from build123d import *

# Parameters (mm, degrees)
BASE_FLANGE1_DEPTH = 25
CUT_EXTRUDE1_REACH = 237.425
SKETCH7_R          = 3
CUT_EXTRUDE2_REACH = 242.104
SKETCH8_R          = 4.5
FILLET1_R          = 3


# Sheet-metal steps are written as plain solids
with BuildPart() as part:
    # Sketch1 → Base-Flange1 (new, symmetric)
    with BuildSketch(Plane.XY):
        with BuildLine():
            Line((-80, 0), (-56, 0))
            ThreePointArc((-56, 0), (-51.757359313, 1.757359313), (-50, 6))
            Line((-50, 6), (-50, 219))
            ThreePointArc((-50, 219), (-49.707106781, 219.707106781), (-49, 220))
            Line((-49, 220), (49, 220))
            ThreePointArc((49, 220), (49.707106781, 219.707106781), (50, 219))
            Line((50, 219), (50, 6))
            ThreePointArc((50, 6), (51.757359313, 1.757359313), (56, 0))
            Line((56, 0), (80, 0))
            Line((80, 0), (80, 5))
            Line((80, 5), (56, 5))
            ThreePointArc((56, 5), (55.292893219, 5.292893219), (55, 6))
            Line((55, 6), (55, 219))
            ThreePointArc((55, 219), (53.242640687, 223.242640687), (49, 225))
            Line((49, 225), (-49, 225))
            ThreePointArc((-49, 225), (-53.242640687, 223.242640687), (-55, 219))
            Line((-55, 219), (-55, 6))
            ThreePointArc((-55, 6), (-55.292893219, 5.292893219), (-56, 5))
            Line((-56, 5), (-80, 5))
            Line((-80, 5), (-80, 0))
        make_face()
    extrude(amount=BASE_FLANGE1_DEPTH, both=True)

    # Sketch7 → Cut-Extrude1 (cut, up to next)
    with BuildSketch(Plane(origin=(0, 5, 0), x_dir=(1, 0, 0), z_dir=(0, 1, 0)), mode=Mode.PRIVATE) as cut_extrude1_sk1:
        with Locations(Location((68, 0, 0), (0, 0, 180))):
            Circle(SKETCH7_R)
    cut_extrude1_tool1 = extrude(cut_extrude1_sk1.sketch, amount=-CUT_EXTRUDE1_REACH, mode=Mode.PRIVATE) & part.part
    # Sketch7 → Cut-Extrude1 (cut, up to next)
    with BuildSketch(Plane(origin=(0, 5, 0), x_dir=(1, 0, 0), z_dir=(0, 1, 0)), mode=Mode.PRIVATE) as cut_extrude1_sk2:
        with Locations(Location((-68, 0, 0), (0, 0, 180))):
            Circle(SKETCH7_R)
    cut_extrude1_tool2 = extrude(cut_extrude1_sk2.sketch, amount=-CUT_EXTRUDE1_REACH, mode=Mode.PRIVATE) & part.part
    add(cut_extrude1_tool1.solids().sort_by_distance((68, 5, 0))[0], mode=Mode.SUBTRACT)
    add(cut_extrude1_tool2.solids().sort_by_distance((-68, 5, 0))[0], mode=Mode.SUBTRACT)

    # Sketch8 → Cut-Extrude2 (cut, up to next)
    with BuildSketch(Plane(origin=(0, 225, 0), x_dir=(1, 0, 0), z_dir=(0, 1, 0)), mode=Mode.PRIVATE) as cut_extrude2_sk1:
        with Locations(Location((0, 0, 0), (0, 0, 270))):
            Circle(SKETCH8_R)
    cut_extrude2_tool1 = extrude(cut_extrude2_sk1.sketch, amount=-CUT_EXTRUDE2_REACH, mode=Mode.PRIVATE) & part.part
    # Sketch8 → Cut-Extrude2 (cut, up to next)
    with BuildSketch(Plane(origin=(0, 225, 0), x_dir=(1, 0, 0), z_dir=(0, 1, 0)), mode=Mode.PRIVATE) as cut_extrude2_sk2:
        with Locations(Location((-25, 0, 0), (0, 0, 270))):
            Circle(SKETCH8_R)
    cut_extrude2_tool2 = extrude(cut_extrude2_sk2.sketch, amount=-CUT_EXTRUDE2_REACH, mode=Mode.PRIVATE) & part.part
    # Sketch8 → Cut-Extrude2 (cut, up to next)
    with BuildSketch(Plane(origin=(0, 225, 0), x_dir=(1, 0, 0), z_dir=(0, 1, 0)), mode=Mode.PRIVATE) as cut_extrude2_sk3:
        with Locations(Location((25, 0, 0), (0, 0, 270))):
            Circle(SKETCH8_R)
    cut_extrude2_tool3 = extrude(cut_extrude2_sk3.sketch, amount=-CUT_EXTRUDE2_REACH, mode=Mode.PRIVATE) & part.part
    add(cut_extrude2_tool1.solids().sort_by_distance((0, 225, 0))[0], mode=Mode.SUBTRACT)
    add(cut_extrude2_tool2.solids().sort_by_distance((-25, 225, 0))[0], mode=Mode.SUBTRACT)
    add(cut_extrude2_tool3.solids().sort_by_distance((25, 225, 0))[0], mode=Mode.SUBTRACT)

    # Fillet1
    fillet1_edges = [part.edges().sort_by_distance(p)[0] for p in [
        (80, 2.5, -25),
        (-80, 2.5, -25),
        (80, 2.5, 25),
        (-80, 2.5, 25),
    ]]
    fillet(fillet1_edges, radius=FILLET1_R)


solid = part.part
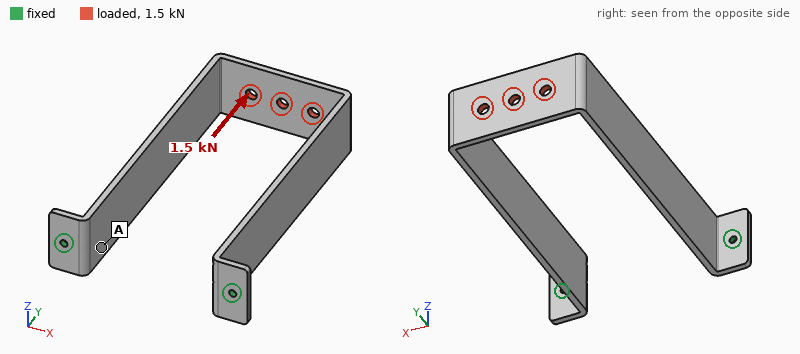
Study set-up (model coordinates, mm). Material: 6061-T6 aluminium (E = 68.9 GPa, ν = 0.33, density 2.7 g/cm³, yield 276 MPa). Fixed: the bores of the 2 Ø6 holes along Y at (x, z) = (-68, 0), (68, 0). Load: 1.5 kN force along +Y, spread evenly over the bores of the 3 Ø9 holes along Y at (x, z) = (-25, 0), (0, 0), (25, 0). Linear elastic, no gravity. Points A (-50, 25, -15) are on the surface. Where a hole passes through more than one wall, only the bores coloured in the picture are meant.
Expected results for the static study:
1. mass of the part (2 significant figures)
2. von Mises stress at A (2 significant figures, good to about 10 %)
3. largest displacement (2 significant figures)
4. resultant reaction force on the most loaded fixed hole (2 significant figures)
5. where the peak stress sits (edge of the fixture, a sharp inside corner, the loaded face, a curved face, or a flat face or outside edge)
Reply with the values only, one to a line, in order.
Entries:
400 g
14 MPa
0.54 mm
750 N
the loaded face
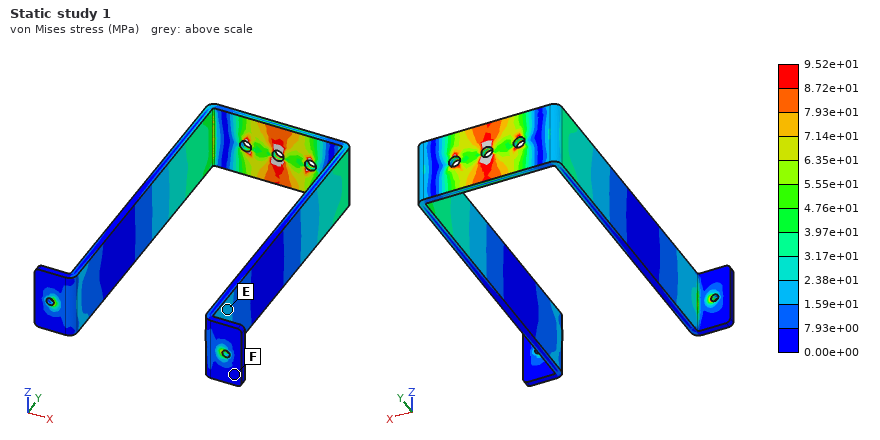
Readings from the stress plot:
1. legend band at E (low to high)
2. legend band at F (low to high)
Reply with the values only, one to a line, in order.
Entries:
1.59e+01 to 2.38e+01 MPa
0.00e+00 to 7.93e+00 MPa
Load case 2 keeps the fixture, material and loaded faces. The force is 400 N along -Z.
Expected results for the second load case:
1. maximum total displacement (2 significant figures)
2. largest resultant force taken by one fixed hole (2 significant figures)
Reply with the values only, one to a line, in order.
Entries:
3.1 mm
200 N
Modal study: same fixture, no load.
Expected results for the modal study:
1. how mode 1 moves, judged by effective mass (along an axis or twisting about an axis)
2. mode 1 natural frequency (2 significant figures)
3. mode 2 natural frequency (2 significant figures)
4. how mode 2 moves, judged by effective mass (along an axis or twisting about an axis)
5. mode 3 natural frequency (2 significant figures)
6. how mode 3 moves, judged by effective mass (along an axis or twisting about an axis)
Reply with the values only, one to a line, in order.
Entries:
along X
93 Hz
140 Hz
along Z
250 Hz
twisting about Y
